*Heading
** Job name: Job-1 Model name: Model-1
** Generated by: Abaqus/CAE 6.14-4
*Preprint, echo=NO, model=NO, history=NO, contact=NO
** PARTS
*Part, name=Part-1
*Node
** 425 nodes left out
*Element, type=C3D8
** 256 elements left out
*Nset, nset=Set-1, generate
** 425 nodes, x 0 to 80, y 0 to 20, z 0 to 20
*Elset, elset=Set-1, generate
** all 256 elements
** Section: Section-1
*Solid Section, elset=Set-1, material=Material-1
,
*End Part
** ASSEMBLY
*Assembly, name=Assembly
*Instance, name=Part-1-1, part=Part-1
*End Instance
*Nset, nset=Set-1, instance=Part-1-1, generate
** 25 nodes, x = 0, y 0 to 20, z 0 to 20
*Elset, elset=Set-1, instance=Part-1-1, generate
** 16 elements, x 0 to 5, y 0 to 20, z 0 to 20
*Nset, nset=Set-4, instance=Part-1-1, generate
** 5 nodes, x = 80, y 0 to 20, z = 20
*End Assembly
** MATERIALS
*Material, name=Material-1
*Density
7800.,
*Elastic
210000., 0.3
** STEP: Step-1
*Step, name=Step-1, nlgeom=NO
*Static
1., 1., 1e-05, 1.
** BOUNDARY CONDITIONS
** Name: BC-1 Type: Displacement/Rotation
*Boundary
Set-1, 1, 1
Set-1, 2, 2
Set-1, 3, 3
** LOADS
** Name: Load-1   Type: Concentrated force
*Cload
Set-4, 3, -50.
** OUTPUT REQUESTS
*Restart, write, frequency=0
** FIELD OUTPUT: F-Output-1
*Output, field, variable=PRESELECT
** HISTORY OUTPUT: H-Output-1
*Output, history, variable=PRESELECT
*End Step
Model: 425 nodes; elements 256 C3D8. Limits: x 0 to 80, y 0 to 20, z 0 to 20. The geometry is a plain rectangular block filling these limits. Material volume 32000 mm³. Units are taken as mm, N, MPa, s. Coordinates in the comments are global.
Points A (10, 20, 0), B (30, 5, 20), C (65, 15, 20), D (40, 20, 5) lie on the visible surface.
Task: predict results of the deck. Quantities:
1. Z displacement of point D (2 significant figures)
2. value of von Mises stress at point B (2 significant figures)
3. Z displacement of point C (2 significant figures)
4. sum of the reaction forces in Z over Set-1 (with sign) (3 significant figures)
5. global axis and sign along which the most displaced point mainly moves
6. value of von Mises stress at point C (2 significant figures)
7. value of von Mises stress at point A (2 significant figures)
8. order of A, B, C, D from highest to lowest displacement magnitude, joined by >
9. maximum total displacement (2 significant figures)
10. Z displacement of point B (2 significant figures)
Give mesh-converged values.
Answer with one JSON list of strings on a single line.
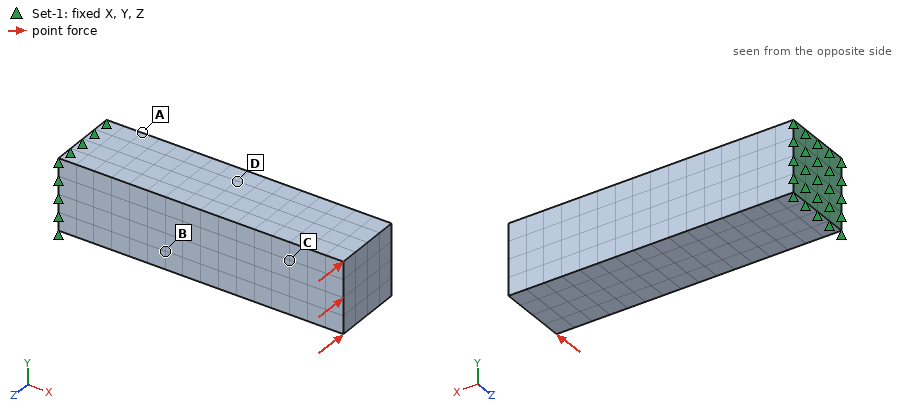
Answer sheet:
["-0.0049 mm", "9.4 MPa", "-0.011 mm", "250 N", "-Z", "3.0 MPa", "12 MPa", "C > D > B > A", "0.017 mm", "-0.0030 mm"]
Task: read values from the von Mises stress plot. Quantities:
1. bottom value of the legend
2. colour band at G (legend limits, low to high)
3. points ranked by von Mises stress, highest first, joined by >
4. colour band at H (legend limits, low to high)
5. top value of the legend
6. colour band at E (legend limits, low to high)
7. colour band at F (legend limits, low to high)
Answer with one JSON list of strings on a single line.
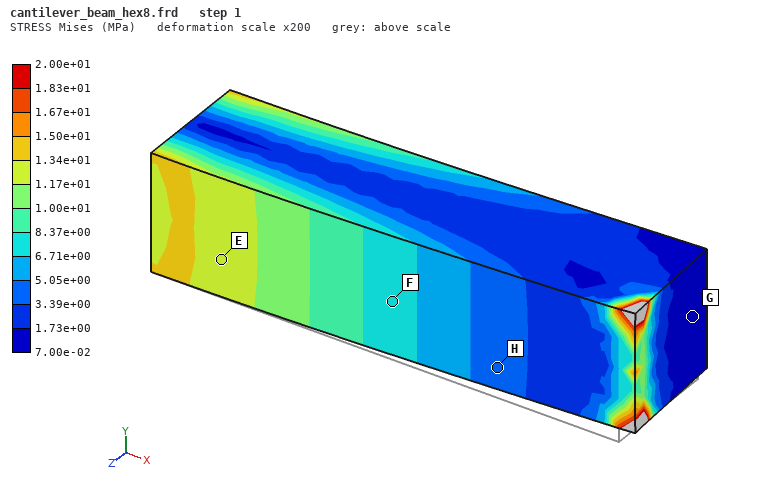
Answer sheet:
["7.00e-02 MPa", "7.00e-02 to 1.73e+00 MPa", "E > F > H > G", "3.39e+00 to 5.05e+00 MPa", "2.00e+01 MPa", "1.17e+01 to 1.34e+01 MPa", "6.71e+00 to 8.37e+00 MPa"]
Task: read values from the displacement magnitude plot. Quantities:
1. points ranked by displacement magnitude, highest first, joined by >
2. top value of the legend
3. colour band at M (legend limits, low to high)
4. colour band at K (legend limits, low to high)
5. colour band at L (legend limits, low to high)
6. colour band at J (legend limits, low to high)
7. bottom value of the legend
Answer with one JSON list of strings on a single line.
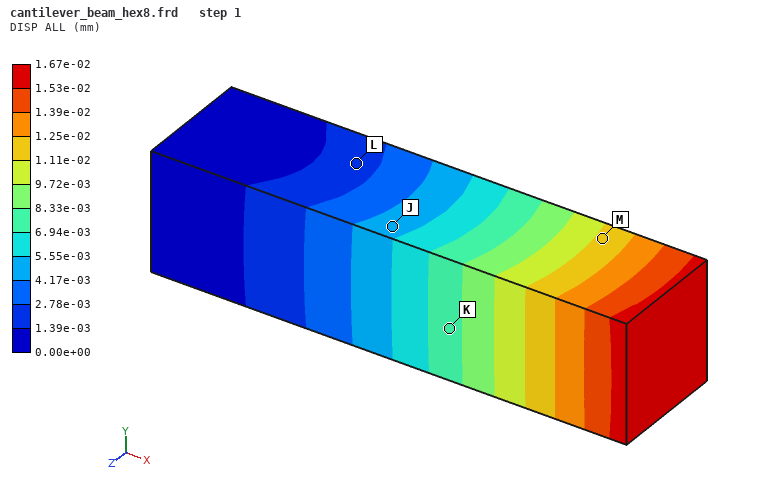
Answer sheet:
["M > K > J > L", "1.67e-02 mm", "1.11e-02 to 1.25e-02 mm", "6.94e-03 to 8.33e-03 mm", "1.39e-03 to 2.78e-03 mm", "4.17e-03 to 5.55e-03 mm", "0.00e+00 mm"]
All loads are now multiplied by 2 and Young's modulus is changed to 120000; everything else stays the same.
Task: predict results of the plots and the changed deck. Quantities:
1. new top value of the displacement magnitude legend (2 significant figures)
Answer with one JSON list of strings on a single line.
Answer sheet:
["0.058 mm"]
